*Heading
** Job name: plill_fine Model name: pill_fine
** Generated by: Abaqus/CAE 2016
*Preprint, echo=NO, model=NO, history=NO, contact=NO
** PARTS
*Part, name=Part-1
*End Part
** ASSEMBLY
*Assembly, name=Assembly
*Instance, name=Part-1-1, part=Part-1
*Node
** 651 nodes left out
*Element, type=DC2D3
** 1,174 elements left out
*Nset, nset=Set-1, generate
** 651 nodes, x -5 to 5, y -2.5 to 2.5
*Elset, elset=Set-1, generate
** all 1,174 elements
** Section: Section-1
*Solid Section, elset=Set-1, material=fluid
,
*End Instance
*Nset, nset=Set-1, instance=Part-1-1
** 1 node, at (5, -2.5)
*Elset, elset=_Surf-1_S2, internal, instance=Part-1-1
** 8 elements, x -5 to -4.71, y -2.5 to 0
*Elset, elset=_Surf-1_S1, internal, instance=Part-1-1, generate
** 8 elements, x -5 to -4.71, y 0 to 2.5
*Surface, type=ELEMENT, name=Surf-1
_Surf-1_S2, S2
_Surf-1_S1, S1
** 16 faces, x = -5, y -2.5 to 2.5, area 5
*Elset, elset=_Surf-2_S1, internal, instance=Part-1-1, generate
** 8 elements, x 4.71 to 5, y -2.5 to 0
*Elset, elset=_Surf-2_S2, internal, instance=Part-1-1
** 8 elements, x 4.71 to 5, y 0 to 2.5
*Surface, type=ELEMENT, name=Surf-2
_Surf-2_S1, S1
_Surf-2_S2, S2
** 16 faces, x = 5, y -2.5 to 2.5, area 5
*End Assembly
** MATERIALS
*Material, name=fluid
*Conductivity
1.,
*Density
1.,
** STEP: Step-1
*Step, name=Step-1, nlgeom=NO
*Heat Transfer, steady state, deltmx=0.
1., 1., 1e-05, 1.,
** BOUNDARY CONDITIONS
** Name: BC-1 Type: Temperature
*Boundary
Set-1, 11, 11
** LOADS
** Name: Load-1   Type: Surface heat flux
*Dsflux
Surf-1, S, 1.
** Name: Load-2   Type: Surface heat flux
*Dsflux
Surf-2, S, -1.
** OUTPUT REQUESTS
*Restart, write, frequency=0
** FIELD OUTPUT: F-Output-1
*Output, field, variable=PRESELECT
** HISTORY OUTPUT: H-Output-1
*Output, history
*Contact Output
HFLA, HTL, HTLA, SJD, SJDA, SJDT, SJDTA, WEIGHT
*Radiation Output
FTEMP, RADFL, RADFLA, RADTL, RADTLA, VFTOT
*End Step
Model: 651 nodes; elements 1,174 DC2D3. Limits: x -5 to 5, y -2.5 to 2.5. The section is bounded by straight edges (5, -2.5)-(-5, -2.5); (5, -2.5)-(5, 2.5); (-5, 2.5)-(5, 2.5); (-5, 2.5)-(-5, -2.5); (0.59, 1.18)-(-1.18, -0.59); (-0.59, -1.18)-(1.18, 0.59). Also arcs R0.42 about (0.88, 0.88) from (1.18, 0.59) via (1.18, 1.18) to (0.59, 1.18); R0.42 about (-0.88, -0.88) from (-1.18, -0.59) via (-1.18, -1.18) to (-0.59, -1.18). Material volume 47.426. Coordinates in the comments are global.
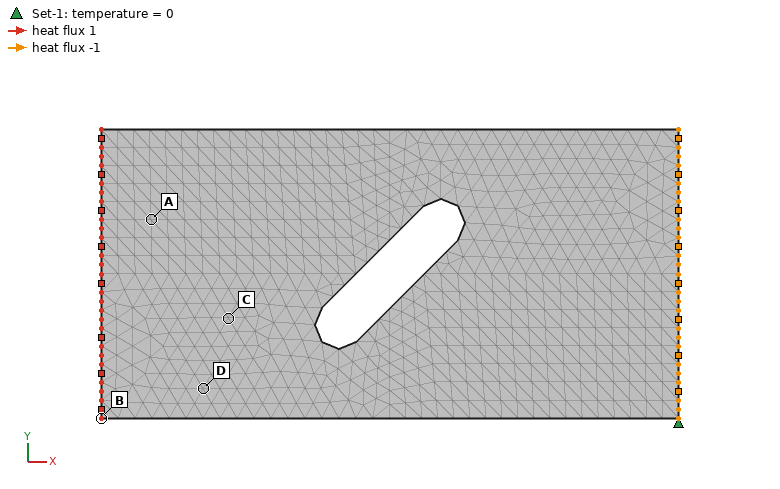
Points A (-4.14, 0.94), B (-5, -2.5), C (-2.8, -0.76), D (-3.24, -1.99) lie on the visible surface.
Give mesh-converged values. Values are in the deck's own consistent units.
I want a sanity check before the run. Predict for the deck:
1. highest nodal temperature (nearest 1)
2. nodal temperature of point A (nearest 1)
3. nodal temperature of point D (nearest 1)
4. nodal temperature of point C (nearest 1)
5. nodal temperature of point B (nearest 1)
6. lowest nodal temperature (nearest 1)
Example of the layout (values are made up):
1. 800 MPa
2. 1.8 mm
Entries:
1. 12
2. 11
3. 10
4. 10
5. 12
6. 0
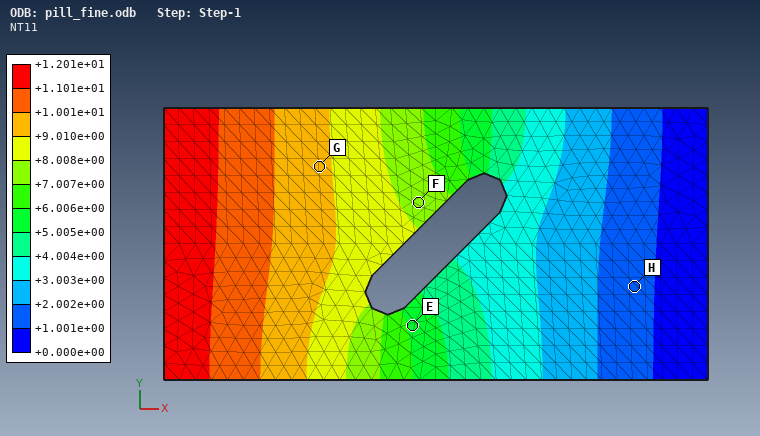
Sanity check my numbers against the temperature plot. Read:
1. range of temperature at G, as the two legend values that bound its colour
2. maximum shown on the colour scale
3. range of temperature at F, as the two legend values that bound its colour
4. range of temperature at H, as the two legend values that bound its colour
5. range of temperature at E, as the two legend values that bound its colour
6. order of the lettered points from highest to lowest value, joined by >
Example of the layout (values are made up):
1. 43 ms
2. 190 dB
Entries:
1. +9.010e+00 to +1.001e+01
2. +1.201e+01
3. +7.007e+00 to +8.008e+00
4. +1.001e+00 to +2.002e+00
5. +5.005e+00 to +6.006e+00
6. G > F > E > H
